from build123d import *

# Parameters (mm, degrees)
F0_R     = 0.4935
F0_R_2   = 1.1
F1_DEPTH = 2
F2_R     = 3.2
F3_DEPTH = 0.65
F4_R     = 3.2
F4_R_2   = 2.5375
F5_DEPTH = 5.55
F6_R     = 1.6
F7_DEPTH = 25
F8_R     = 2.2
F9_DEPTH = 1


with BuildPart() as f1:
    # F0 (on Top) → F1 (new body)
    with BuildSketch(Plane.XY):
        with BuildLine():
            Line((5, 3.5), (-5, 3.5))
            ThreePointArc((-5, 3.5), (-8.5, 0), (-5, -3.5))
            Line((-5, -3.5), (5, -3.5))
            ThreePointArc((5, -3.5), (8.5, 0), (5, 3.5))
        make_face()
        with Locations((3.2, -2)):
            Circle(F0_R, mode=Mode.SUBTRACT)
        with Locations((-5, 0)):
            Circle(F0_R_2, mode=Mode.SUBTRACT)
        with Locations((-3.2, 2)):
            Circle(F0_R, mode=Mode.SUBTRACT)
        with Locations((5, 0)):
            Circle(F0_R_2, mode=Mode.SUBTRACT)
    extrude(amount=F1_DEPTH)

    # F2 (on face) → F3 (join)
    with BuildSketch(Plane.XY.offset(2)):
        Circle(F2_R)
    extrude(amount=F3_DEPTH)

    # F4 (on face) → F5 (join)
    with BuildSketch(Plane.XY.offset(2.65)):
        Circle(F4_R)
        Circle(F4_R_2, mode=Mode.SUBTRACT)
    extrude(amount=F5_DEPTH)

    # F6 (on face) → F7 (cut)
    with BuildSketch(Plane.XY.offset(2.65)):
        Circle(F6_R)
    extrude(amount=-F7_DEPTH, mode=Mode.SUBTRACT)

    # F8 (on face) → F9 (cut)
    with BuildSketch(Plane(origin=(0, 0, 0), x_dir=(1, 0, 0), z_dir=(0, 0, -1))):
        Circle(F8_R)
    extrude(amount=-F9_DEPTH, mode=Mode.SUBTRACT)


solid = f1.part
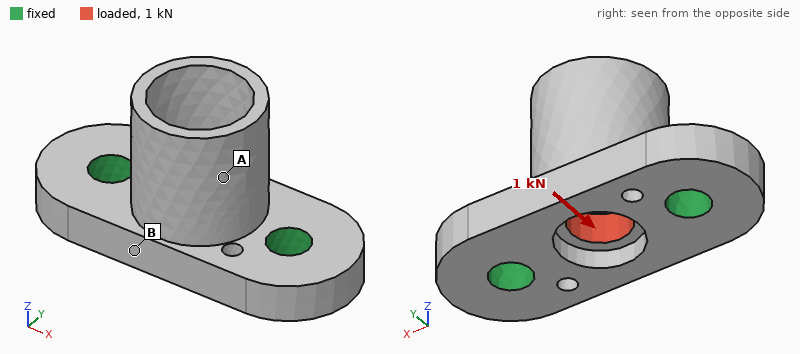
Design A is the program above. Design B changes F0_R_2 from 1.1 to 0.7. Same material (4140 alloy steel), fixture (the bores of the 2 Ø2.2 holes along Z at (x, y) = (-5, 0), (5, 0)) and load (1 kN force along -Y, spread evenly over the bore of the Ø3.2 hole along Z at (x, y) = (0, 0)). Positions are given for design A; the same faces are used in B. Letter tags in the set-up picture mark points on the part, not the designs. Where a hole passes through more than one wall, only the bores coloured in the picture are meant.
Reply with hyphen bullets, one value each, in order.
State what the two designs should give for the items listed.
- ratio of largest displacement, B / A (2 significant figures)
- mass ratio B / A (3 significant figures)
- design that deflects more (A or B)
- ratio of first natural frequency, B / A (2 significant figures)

- 1.4
- 1.04
- B
- 0.87
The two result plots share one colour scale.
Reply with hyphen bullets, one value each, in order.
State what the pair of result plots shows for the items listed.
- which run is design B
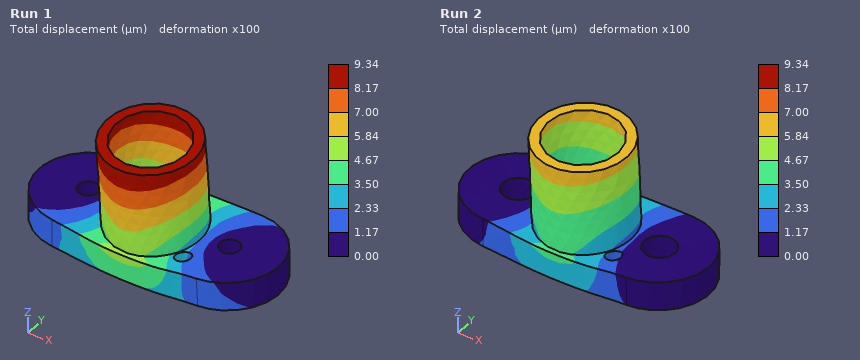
- Run 1
